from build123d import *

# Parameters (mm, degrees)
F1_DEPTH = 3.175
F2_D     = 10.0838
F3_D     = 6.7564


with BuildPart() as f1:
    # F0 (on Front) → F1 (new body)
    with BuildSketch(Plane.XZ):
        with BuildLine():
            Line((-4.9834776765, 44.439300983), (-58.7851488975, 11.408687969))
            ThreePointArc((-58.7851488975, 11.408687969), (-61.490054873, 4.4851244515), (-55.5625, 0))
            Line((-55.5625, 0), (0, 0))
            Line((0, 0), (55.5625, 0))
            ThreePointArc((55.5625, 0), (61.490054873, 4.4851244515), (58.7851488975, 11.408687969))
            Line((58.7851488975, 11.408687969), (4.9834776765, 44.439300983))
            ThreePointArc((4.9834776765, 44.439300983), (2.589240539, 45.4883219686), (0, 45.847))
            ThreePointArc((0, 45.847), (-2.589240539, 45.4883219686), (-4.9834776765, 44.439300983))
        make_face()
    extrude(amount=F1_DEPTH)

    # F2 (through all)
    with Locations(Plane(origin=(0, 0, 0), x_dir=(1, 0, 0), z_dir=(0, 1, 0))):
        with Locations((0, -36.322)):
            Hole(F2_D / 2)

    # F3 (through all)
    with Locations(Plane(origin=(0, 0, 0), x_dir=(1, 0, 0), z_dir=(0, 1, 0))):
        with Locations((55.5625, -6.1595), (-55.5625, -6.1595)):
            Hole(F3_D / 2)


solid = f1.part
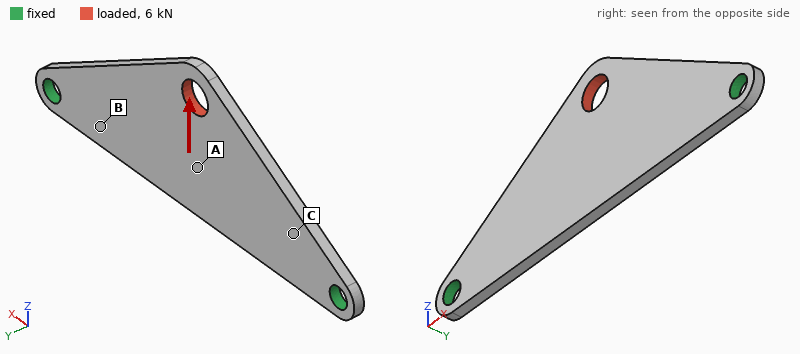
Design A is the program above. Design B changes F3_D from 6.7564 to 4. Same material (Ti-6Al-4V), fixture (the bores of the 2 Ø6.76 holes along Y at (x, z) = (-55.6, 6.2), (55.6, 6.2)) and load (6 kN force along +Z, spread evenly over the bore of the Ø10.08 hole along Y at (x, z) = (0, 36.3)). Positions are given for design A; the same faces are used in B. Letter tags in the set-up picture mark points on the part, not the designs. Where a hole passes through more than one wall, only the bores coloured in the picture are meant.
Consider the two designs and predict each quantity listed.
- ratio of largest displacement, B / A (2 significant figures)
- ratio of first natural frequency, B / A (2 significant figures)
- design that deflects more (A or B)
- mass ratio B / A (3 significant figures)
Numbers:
1.1
0.93
B
1.01
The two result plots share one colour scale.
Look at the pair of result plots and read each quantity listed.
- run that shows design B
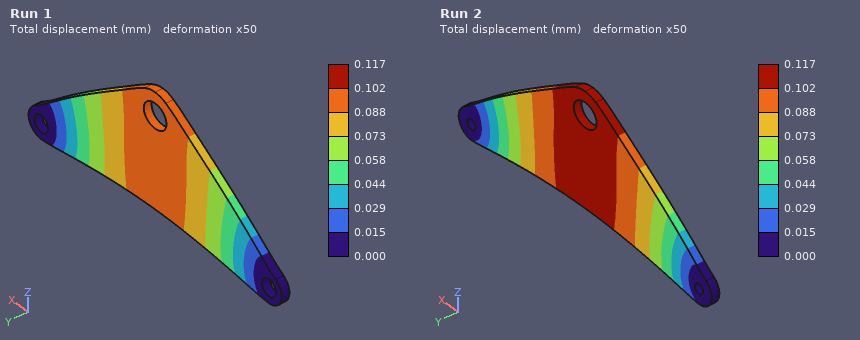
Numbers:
Run 2
